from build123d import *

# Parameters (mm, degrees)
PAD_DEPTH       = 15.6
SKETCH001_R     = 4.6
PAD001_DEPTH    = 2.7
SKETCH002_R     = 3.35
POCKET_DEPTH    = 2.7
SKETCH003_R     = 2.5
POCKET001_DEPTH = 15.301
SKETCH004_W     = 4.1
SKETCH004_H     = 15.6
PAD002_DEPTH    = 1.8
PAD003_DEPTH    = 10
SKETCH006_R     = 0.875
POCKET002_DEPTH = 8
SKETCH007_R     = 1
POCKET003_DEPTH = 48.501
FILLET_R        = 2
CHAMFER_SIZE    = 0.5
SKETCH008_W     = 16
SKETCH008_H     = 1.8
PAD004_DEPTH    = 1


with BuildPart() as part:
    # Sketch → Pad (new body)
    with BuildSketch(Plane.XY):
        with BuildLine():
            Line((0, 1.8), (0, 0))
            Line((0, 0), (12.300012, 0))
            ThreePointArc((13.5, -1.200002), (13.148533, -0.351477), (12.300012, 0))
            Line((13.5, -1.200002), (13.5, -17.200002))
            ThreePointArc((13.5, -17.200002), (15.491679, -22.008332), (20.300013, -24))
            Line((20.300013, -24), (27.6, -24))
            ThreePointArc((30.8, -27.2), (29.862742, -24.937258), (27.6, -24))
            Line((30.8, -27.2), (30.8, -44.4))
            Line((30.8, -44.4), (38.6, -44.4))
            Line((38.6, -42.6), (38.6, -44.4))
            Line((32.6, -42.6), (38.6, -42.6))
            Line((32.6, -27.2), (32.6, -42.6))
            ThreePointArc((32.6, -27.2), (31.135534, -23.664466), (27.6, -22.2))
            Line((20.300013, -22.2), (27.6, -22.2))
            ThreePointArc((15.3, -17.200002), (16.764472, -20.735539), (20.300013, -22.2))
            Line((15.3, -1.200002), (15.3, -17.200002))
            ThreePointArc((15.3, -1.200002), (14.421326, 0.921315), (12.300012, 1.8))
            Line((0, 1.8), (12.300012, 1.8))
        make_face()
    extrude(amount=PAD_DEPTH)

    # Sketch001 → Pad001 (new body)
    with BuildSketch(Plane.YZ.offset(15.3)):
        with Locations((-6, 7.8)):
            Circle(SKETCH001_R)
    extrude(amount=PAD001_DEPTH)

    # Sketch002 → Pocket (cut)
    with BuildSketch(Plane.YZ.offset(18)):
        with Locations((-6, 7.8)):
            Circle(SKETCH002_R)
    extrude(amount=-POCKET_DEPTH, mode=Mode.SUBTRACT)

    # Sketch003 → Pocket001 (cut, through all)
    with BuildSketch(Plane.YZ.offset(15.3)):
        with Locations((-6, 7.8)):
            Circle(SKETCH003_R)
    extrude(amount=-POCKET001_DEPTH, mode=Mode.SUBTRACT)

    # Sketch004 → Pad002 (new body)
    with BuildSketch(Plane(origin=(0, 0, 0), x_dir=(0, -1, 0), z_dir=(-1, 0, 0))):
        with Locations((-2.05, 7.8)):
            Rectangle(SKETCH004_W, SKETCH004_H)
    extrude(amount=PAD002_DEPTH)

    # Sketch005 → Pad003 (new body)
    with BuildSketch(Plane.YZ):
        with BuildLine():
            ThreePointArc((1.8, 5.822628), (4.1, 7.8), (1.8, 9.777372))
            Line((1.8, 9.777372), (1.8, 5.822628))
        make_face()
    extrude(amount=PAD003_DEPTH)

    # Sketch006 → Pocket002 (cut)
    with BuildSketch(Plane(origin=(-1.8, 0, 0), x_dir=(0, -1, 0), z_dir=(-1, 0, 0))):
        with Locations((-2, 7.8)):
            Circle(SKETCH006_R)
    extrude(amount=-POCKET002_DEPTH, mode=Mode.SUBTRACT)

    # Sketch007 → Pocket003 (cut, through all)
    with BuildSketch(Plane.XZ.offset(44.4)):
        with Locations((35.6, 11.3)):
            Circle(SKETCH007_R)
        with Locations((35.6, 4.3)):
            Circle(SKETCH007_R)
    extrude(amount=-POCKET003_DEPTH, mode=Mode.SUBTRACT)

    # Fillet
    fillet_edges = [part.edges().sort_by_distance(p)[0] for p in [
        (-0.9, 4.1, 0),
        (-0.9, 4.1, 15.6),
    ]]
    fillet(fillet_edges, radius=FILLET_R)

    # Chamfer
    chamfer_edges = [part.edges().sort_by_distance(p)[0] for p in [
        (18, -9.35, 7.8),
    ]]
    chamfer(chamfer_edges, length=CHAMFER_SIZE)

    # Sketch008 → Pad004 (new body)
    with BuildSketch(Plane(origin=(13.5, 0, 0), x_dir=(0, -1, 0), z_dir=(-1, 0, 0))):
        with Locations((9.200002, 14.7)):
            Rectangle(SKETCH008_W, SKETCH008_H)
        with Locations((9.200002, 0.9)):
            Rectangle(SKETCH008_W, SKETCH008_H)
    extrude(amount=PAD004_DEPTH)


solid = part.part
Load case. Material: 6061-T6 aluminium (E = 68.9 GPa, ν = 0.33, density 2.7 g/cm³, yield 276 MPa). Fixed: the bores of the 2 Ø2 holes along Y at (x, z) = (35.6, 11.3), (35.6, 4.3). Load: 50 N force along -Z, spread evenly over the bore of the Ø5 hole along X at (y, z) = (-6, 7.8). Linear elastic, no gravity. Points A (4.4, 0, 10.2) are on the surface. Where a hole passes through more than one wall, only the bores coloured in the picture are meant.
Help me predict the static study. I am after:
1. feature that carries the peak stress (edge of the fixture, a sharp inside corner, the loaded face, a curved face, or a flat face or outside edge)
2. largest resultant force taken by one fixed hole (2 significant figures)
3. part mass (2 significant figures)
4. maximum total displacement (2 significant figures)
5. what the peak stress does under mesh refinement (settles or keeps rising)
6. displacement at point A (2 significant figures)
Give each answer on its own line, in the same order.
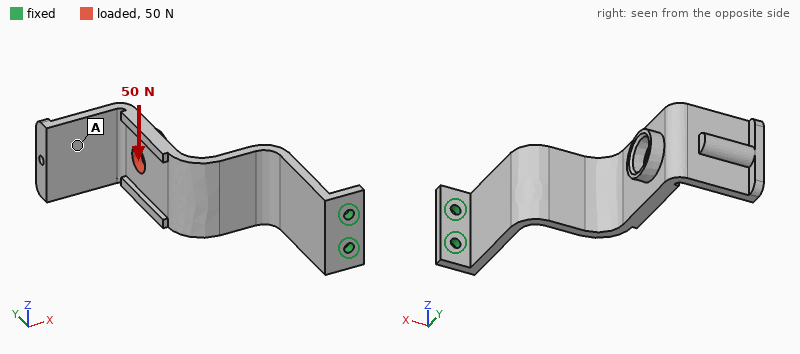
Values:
edge of the fixture
240 N
6.6 g
0.76 mm
keeps rising
0.65 mm
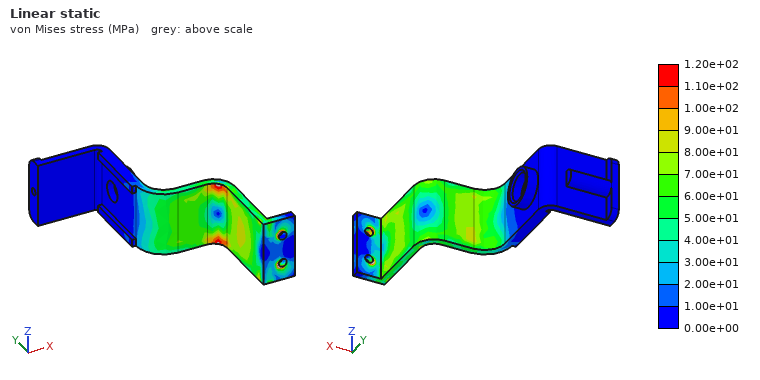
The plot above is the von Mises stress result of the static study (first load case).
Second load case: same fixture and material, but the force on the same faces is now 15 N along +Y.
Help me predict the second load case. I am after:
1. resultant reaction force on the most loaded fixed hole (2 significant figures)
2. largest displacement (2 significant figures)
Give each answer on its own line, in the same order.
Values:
9.4 N
0.70 mm
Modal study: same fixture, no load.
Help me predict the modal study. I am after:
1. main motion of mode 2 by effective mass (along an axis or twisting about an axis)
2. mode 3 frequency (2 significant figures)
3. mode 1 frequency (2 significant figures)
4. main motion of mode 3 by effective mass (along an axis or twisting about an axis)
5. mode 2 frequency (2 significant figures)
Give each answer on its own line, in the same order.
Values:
along Z
1900 Hz
300 Hz
along X
730 Hz
